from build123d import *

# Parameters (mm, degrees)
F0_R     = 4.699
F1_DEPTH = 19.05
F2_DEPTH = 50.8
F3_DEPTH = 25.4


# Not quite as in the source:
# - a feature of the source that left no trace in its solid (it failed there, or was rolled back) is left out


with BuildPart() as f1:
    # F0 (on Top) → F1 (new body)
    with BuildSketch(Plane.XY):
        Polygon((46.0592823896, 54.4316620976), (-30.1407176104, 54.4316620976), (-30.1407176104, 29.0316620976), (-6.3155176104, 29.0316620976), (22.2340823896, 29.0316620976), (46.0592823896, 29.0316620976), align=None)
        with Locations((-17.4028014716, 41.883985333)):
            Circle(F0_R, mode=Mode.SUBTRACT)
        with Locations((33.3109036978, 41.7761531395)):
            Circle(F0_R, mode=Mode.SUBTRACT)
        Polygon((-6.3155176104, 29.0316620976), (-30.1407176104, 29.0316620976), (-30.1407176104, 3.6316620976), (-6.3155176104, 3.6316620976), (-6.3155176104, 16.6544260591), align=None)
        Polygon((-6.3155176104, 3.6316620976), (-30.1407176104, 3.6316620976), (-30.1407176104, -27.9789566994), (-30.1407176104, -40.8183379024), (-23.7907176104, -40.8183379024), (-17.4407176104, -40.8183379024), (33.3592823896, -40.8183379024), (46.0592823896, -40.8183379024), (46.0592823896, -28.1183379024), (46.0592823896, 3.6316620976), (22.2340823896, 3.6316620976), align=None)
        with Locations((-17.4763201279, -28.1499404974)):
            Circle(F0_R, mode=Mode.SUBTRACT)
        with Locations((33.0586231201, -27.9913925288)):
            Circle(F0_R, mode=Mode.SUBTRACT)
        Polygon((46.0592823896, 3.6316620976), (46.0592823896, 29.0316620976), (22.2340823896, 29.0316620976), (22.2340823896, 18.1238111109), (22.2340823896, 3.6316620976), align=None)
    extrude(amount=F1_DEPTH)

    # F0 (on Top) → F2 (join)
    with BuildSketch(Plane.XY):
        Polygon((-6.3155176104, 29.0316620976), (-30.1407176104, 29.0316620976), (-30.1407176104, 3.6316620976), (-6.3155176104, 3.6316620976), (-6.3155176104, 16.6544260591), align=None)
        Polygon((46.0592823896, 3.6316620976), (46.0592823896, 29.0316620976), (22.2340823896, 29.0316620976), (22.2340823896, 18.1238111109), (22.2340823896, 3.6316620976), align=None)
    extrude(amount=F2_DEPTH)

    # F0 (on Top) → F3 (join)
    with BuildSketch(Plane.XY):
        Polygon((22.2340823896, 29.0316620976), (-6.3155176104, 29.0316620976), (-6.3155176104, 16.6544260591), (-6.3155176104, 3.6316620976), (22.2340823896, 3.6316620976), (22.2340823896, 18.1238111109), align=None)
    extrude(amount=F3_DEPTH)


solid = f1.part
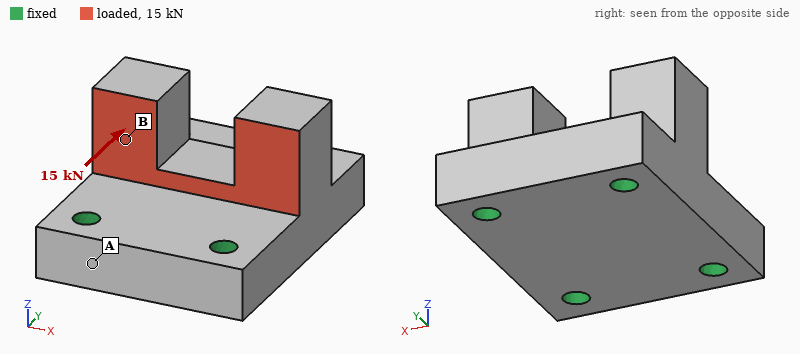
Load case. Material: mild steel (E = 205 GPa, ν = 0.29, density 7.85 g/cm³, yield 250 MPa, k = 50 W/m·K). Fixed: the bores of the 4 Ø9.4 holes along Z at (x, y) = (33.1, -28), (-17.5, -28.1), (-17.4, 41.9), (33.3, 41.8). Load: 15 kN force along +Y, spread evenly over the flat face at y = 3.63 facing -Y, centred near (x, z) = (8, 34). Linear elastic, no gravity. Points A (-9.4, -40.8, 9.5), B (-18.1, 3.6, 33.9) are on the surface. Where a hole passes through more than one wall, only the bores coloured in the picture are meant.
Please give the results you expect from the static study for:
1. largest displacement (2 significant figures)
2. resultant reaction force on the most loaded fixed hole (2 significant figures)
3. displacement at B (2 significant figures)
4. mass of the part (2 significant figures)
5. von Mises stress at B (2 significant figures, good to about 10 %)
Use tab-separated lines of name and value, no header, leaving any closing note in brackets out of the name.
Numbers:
largest displacement	16 µm
resultant reaction force on the most loaded fixed hole	5.4 kN
displacement at B	9.9 µm
mass of the part	1.4 kg
von Mises stress at B	16 MPa
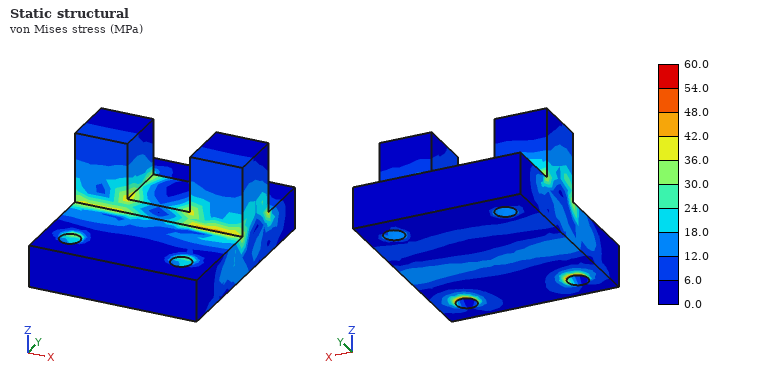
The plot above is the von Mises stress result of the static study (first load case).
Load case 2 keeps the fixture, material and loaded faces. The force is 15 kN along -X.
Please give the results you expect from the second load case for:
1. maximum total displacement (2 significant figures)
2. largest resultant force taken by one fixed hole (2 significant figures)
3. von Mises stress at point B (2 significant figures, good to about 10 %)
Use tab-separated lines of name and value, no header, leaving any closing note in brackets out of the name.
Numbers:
maximum total displacement	24 µm
largest resultant force taken by one fixed hole	6.6 kN
von Mises stress at point B	46 MPa
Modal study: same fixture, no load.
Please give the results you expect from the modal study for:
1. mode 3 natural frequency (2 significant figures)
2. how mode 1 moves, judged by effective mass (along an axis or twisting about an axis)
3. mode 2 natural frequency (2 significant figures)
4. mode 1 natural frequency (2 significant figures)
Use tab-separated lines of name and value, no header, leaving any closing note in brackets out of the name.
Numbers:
mode 3 natural frequency	9900 Hz
how mode 1 moves, judged by effective mass	along X
mode 2 natural frequency	9300 Hz
mode 1 natural frequency	8600 Hz
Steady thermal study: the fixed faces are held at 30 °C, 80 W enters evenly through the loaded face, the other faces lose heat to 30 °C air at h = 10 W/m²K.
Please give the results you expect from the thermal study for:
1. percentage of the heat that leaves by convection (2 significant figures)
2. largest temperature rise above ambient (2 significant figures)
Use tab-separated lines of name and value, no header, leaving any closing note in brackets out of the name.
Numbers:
percentage of the heat that leaves by convection	3.6 %
largest temperature rise above ambient	44 K
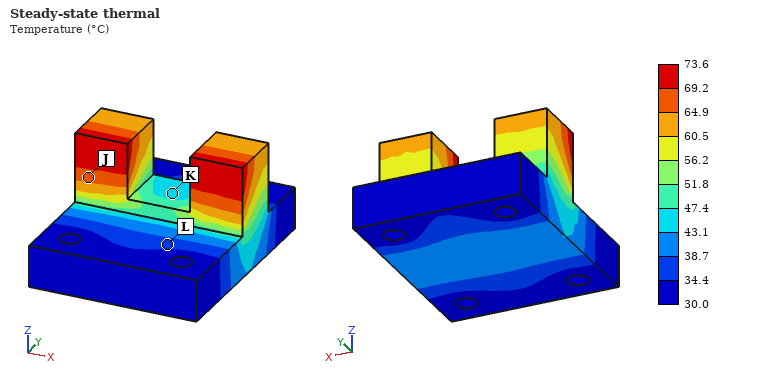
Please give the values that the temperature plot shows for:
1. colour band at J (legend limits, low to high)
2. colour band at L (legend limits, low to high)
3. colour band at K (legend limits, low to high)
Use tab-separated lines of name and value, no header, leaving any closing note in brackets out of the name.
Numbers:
colour band at J	64.9 to 69.2 °C
colour band at L	34.4 to 38.7 °C
colour band at K	43.1 to 47.4 °C
